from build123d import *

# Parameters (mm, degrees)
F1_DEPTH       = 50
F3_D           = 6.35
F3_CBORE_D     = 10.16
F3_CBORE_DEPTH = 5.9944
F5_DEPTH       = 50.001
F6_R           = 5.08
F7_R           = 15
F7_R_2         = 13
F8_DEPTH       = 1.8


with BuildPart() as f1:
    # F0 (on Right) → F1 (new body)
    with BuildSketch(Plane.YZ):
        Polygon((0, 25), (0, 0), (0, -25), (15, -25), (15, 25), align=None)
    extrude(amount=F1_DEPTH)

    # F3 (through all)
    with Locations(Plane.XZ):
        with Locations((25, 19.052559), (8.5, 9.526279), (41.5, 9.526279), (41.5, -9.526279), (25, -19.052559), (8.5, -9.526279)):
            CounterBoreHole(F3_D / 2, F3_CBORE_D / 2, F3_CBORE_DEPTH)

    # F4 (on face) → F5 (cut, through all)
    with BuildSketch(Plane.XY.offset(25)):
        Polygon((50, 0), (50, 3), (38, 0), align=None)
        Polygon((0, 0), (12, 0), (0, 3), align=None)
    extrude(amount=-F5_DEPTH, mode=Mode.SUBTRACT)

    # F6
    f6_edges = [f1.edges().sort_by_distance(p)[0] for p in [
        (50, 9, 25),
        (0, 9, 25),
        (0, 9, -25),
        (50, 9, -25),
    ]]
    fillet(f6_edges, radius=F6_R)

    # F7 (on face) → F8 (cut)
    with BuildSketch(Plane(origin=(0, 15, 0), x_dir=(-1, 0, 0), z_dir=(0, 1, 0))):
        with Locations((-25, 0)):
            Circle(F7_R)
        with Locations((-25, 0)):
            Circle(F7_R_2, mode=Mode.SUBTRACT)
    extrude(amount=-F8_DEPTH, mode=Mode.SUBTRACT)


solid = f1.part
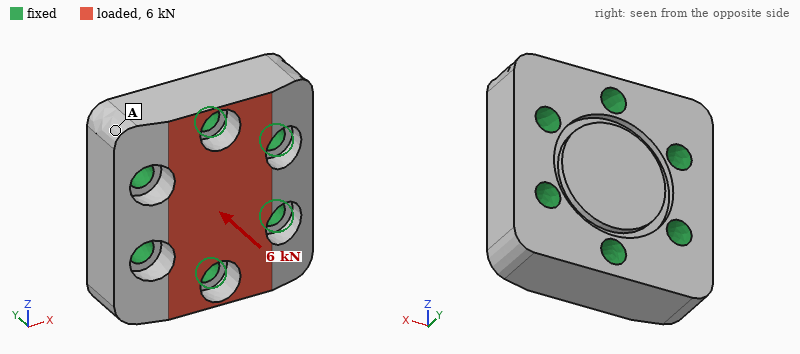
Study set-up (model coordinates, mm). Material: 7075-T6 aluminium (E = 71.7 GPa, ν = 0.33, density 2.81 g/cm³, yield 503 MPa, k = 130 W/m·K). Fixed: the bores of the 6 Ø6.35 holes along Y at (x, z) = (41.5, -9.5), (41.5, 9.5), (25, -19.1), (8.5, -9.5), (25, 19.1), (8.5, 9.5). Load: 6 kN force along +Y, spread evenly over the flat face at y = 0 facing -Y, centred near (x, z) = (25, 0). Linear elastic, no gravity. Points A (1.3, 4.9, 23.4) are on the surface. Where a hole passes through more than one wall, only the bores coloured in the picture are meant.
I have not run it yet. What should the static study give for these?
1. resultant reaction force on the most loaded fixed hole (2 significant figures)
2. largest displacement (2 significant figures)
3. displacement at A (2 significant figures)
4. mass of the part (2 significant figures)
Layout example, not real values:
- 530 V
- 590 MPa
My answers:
- 1.4 kN
- 2.3 µm
- 0.68 µm
- 86 g
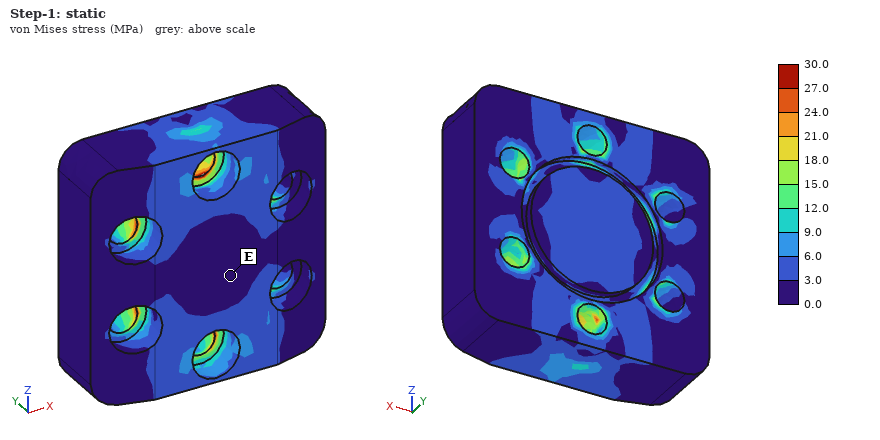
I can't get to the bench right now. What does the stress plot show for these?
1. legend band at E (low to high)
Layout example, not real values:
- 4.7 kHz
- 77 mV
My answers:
- 0.0 to 3.0 MPa
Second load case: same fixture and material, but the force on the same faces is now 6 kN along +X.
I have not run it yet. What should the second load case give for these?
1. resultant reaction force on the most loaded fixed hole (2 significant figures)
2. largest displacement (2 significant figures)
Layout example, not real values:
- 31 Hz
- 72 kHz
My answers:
- 1.3 kN
- 3.0 µm
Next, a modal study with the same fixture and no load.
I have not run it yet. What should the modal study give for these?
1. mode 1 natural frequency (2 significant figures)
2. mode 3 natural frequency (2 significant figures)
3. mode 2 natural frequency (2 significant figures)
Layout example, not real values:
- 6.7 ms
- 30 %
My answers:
- 35 kHz
- 35 kHz
- 35 kHz
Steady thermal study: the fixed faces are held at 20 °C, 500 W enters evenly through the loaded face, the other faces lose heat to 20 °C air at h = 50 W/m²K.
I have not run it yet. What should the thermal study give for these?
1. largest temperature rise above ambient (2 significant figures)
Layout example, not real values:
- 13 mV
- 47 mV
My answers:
- 47 K
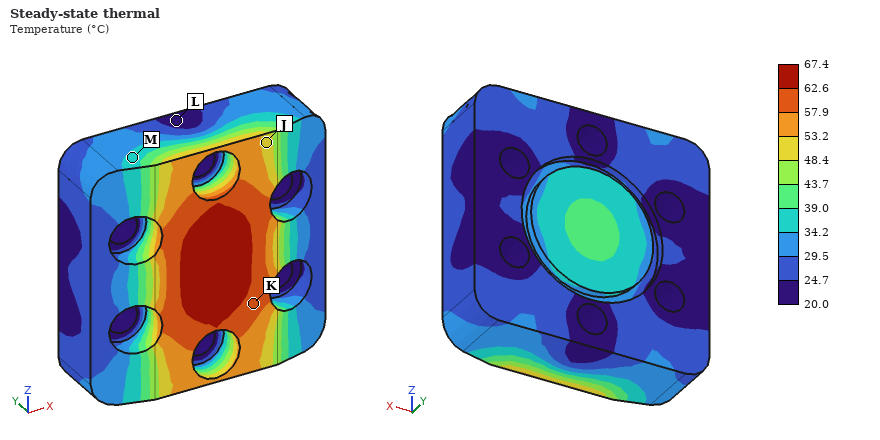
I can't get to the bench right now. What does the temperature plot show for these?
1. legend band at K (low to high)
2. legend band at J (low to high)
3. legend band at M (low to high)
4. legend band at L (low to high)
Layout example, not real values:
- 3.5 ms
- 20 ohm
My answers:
- 57.9 to 62.6 °C
- 48.4 to 53.2 °C
- 34.2 to 39.0 °C
- 20.0 to 24.7 °C
